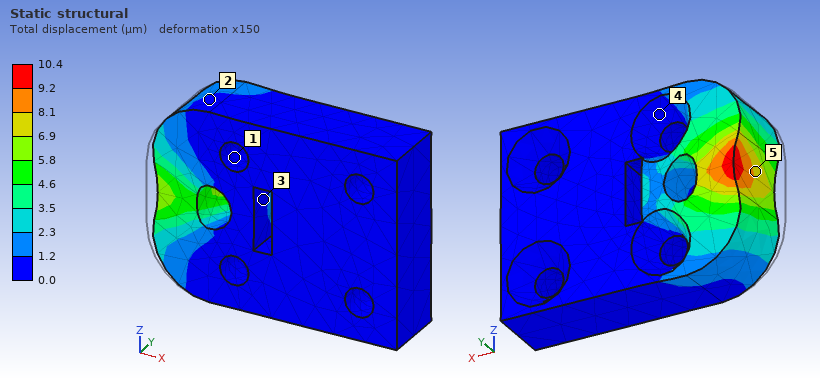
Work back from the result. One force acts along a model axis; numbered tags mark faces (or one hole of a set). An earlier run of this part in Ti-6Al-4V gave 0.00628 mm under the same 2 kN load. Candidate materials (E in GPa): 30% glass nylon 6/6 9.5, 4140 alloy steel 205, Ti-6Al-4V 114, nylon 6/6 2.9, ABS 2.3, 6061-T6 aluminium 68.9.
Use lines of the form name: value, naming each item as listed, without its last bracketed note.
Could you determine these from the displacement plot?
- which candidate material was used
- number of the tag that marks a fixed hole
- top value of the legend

which candidate material was used: 6061-T6 aluminium
number of the tag that marks a fixed hole: 1
top value of the legend: 10.4 µm
